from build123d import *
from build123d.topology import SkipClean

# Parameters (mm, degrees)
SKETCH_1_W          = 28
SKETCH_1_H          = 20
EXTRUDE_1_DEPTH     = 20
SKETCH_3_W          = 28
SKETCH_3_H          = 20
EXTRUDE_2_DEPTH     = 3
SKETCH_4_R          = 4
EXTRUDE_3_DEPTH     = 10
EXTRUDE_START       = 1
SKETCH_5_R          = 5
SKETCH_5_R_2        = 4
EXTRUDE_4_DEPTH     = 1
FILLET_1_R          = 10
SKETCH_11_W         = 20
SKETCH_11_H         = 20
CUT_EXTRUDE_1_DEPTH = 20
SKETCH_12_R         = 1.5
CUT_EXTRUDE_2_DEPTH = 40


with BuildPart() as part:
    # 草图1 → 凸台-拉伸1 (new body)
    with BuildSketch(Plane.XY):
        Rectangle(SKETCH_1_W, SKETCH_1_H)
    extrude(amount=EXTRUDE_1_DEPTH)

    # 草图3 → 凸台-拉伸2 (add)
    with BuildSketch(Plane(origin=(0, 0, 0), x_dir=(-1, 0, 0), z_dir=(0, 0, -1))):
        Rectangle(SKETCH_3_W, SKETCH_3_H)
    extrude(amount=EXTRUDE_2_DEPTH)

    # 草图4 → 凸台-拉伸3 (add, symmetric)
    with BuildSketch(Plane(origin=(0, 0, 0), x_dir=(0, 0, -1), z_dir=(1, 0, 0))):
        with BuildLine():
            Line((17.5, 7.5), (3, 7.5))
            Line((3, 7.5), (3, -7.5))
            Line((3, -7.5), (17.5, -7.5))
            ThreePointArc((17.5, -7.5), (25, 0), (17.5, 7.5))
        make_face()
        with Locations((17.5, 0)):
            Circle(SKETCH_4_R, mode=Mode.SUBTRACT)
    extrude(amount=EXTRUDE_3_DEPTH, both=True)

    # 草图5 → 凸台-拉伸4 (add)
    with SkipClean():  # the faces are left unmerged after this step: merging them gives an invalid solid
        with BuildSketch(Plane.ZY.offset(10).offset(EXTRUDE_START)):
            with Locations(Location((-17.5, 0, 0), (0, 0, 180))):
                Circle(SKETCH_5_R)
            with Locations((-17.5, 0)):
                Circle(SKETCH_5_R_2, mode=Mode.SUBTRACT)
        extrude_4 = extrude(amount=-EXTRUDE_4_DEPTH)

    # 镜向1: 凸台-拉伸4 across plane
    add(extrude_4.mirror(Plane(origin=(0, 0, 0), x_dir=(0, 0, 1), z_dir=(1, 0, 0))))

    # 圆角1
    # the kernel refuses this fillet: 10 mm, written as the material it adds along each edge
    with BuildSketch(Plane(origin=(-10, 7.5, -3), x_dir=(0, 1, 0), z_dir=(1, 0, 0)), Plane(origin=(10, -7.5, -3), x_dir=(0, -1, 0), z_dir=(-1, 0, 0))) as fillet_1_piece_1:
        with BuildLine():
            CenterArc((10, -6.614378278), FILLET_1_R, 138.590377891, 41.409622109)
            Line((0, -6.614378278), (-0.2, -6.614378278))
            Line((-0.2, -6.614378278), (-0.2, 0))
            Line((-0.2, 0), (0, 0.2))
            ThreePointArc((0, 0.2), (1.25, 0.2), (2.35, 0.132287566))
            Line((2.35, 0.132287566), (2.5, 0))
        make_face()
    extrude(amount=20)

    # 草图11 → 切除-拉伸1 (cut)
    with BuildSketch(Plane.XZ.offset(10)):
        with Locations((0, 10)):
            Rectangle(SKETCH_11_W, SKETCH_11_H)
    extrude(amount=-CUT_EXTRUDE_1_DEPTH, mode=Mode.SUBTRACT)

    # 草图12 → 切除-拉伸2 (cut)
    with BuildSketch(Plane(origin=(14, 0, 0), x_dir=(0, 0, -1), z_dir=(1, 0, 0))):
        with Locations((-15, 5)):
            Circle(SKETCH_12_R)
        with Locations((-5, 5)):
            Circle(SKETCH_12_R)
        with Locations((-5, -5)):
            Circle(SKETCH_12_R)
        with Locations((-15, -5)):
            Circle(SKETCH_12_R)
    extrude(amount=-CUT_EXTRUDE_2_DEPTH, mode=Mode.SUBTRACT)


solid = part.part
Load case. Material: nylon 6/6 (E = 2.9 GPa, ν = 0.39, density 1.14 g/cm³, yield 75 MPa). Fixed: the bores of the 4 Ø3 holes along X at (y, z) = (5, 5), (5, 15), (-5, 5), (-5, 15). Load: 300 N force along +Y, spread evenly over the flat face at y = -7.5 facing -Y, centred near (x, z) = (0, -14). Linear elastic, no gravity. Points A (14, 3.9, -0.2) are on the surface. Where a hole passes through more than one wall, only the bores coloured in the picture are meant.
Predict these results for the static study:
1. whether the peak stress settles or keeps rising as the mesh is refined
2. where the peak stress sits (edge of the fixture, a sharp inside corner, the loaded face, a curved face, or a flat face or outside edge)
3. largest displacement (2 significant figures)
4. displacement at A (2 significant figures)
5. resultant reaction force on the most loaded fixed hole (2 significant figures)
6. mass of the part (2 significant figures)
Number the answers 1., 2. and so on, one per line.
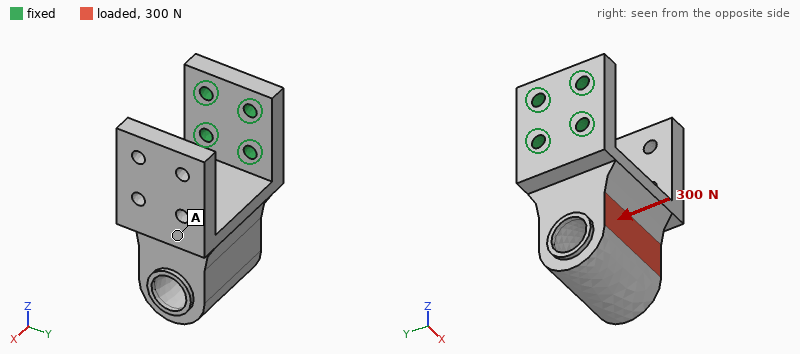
1. keeps rising
2. edge of the fixture
3. 0.58 mm
4. 0.39 mm
5. 490 N
6. 11 g
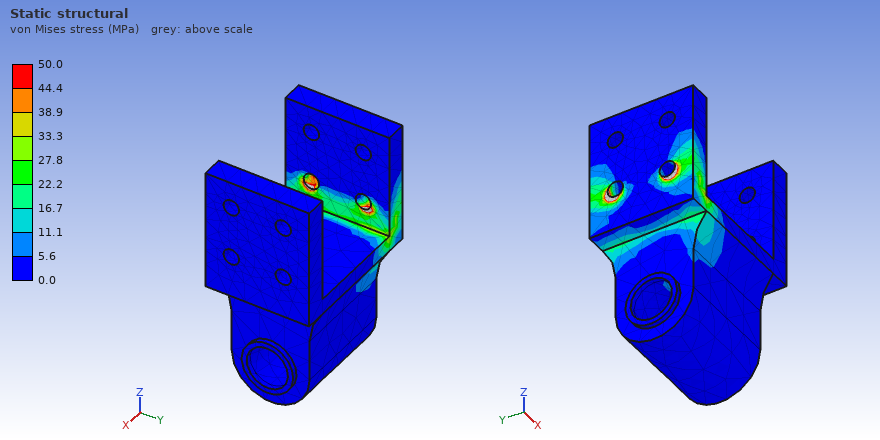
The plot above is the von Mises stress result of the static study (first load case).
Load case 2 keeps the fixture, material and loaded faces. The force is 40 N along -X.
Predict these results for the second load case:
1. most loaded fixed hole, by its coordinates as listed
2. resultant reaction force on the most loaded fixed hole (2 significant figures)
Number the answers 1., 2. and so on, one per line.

1. (-5, 5)
2. 50 N
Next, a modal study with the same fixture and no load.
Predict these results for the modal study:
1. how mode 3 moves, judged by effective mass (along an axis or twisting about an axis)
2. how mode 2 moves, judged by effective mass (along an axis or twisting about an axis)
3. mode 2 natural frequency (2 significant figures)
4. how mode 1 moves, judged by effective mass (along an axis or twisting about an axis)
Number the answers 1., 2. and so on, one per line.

1. along X
2. along Y
3. 1200 Hz
4. along Z
